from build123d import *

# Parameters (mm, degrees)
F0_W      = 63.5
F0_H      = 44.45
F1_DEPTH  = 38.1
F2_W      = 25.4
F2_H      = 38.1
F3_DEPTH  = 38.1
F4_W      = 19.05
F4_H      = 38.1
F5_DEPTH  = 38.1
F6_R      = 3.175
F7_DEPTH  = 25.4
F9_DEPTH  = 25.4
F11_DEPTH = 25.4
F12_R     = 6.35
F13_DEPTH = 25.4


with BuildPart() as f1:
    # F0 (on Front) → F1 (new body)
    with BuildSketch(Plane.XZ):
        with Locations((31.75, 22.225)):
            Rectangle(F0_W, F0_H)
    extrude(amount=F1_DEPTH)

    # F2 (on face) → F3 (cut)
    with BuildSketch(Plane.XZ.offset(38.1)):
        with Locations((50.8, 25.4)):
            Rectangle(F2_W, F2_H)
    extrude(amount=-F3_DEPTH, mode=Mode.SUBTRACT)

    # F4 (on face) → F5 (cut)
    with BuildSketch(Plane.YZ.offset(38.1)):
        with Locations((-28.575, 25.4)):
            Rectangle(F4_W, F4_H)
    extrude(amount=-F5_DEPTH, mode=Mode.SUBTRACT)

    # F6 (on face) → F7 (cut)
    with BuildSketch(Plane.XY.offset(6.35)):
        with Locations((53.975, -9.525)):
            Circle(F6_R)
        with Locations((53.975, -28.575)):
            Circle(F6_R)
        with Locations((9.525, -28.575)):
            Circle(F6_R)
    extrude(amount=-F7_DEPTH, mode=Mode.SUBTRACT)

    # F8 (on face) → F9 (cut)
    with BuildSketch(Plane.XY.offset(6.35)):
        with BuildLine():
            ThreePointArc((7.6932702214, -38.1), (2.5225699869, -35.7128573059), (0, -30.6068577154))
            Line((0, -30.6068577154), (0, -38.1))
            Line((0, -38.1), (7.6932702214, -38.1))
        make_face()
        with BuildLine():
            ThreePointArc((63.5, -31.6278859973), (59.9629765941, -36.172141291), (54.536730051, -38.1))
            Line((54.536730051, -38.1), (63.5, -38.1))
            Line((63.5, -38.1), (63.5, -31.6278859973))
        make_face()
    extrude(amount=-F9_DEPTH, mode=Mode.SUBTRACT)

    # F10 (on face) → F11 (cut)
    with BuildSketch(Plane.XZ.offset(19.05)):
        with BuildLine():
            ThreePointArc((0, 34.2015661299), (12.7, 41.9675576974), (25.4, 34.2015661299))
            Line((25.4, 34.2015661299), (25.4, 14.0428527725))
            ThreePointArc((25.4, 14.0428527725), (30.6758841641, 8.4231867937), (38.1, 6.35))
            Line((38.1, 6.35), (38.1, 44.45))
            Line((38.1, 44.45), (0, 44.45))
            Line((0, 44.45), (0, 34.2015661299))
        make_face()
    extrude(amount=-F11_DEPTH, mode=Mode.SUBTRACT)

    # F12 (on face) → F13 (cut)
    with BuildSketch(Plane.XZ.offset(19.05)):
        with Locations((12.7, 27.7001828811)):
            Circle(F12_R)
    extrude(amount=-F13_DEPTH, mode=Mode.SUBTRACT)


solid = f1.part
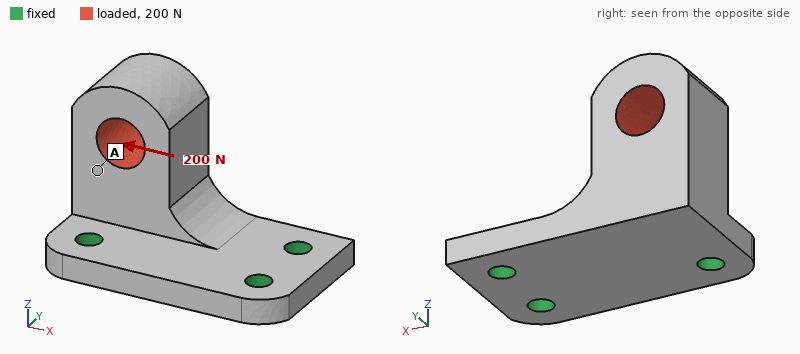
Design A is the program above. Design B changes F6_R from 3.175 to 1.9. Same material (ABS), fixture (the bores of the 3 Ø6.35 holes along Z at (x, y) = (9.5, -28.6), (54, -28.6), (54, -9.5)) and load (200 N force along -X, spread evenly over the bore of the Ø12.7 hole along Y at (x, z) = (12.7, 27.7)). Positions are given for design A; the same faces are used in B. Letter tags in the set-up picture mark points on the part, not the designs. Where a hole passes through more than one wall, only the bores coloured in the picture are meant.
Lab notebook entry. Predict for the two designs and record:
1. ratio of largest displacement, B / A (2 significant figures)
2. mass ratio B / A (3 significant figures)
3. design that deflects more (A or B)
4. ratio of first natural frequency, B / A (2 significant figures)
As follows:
1.2
1.01
B
0.91
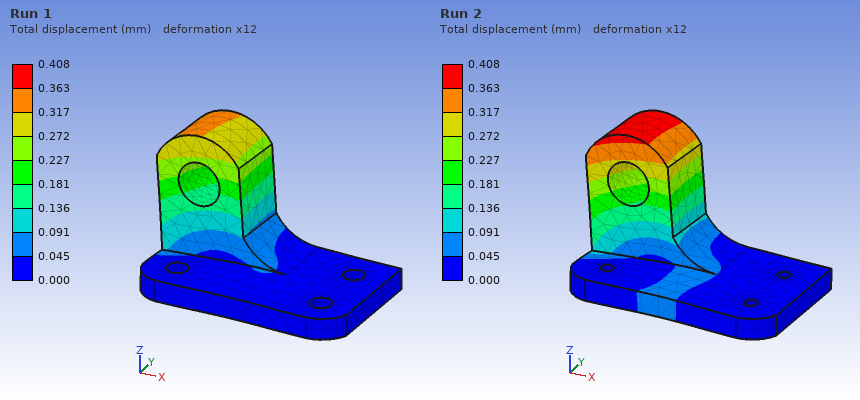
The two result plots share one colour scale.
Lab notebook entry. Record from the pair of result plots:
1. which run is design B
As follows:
Run 2
